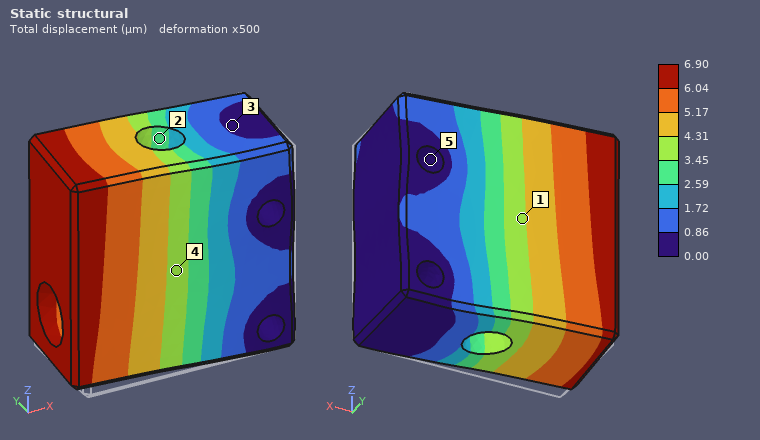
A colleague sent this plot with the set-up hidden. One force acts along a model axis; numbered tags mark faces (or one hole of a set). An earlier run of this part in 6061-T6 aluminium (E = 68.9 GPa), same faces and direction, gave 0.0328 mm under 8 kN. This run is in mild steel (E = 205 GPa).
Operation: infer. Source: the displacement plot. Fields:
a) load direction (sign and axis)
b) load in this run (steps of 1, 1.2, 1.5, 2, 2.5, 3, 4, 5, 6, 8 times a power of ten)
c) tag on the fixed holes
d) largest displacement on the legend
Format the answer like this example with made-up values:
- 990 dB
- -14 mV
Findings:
- +Y
- 5 kN
- 5
- 6.90 µm
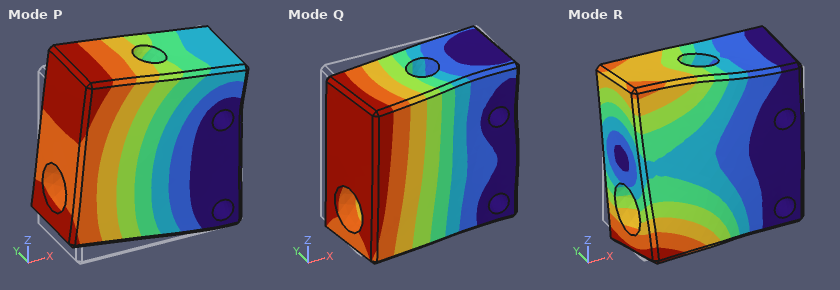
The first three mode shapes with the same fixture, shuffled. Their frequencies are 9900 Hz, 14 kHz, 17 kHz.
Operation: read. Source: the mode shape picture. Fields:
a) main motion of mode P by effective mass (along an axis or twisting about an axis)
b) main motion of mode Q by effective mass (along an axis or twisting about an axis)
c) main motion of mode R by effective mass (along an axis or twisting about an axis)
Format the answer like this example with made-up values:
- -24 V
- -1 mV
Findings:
- along Z
- along Y
- twisting about X
